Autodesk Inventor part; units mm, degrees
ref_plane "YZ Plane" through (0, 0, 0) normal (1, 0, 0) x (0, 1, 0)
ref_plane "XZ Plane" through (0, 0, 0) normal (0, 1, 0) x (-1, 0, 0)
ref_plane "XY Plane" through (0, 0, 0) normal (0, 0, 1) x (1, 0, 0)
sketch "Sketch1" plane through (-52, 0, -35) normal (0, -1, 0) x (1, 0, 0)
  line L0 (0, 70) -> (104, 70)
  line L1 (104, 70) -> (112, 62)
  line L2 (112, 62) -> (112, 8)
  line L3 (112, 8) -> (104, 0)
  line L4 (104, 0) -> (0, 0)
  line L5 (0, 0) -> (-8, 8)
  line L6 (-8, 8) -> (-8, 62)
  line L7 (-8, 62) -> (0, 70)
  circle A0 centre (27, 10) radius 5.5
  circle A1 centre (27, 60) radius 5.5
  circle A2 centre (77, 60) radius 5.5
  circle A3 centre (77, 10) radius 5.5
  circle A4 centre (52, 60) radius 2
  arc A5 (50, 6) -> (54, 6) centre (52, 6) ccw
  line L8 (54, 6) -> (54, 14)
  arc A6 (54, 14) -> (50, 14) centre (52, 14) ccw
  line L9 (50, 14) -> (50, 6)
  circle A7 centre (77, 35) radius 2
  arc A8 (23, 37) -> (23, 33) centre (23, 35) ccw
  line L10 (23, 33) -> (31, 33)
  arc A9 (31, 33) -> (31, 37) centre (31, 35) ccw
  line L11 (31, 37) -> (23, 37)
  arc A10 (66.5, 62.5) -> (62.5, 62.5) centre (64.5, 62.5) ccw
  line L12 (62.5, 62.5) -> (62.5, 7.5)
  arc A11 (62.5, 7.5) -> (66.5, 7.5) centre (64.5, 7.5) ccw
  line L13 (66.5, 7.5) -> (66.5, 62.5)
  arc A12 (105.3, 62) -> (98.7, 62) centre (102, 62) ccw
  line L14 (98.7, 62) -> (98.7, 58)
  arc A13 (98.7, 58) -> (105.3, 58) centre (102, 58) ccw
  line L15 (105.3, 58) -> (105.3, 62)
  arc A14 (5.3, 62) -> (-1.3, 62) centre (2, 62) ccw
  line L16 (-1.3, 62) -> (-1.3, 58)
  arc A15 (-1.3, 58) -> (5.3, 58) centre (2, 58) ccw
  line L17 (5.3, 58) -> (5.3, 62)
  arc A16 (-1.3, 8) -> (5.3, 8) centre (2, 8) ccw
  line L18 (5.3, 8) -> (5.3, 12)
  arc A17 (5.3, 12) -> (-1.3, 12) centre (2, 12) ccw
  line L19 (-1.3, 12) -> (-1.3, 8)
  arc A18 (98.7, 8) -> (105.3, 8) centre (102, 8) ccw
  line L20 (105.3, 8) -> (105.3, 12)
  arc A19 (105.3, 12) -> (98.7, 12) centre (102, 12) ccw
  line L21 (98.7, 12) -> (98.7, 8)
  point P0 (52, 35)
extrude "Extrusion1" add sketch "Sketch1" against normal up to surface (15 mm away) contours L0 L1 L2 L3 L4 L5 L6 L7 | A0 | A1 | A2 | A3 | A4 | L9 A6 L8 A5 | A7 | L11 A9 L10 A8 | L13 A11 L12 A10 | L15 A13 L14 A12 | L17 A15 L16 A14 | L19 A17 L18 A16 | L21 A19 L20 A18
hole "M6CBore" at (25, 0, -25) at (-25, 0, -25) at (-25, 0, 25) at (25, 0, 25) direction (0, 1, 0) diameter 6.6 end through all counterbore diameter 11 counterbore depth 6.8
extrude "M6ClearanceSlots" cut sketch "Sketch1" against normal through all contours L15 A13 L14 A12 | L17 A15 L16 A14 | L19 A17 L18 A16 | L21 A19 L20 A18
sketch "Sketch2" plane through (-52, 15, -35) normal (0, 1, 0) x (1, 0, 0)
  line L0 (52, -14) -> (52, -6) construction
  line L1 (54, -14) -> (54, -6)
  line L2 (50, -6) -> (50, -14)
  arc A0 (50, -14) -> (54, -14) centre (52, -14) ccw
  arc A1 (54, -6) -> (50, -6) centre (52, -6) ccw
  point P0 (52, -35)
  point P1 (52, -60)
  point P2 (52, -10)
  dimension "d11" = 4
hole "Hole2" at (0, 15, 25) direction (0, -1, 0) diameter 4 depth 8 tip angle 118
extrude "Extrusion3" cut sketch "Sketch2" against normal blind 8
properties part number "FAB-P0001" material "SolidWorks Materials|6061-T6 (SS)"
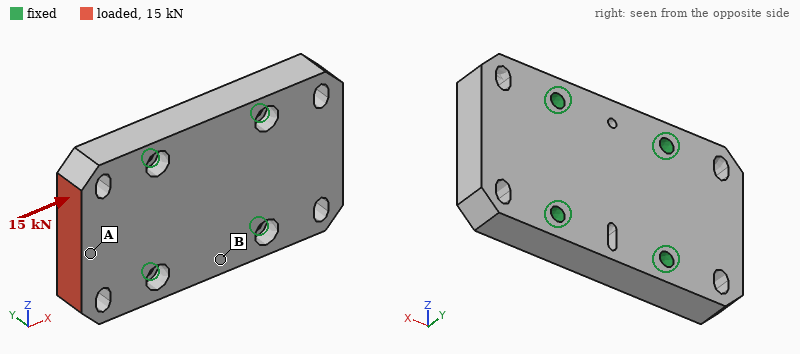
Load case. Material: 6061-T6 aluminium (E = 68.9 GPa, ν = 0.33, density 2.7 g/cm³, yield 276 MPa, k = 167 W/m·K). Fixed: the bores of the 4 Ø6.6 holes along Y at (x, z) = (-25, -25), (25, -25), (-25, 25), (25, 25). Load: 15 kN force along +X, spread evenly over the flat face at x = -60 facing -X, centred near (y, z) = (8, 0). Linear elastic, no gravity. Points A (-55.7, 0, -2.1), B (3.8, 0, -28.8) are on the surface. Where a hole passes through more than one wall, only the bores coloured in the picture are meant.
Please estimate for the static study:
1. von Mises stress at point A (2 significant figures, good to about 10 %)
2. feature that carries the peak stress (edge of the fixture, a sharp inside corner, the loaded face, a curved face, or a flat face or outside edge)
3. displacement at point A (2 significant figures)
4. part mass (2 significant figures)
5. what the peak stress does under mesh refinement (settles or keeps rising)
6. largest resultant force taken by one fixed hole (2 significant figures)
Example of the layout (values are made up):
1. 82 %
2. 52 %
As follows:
1. 17 MPa
2. edge of the fixture
3. 20 µm
4. 310 g
5. keeps rising
6. 5.7 kN
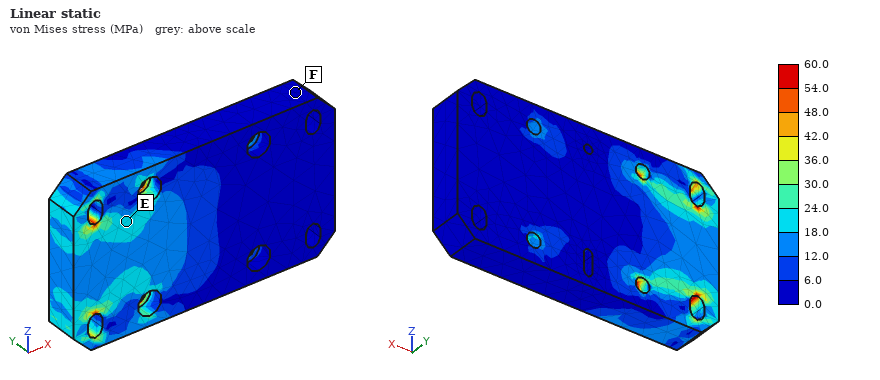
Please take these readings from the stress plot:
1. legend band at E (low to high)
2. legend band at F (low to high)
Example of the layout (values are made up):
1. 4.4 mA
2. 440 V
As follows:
1. 18.0 to 24.0 MPa
2. 0.0 to 6.0 MPa
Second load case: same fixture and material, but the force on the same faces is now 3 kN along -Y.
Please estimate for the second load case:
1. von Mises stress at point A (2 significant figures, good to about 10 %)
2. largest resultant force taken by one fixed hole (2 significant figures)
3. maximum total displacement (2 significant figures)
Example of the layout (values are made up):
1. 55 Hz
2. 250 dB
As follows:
1. 16 MPa
2. 2.6 kN
3. 77 µm
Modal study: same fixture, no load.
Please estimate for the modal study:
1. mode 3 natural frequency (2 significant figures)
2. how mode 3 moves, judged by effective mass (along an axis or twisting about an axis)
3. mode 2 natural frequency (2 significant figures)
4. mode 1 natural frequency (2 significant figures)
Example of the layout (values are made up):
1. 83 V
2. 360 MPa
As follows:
1. 12 kHz
2. twisting about X
3. 6400 Hz
4. 6400 Hz
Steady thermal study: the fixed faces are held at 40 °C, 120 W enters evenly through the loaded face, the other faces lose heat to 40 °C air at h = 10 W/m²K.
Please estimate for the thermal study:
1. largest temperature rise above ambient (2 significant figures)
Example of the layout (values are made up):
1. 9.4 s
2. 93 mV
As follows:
1. 35 K
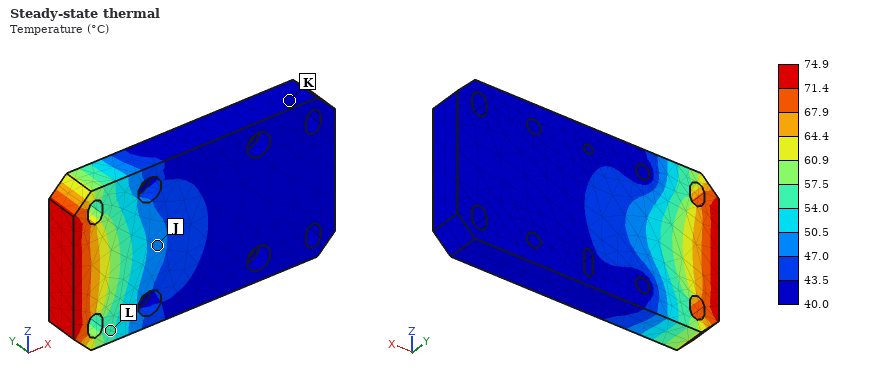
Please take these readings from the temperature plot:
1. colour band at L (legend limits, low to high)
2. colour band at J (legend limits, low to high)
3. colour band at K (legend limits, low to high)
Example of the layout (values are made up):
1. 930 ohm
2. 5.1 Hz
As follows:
1. 54.0 to 57.5 °C
2. 47.0 to 50.5 °C
3. 40.0 to 43.5 °C
